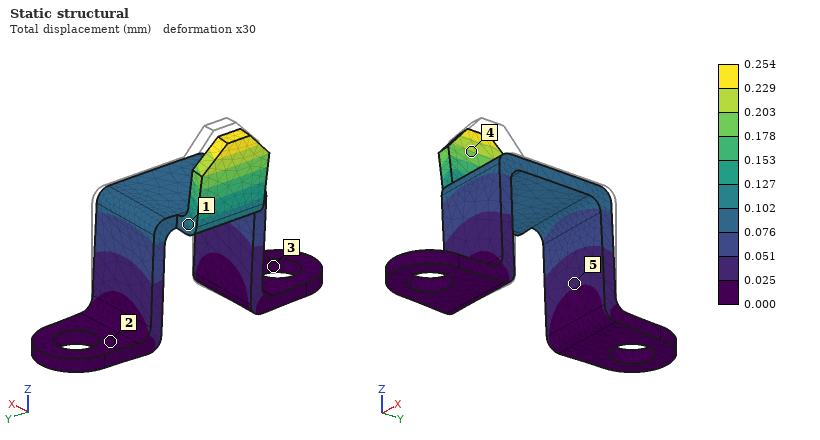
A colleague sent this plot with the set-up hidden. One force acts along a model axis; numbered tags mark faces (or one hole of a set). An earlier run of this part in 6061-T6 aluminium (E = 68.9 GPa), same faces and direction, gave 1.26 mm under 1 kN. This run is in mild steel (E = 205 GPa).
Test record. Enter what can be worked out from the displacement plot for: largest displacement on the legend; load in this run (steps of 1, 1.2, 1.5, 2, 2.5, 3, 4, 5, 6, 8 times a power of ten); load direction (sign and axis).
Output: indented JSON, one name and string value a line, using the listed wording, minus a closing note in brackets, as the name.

{
  "largest displacement on the legend": "0.254 mm",
  "load in this run": "600 N",
  "load direction": "-X"
}
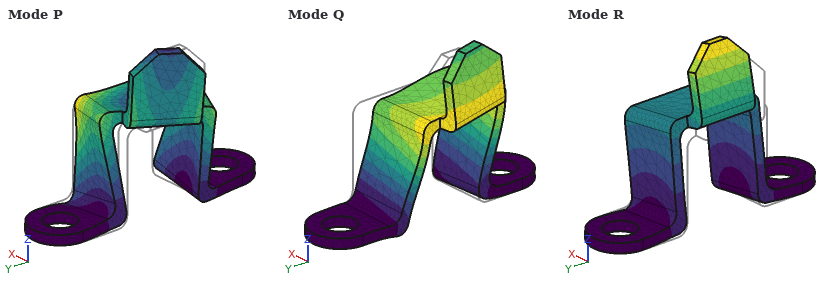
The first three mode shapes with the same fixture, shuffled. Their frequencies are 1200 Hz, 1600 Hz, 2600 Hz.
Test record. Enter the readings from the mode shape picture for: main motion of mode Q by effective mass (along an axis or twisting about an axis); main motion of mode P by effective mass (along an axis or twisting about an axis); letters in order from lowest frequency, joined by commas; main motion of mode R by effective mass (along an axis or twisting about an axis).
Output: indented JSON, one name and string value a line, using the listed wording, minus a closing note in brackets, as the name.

{
  "main motion of mode Q by effective mass": "along Y",
  "main motion of mode P by effective mass": "twisting about Z",
  "letters in order from lowest frequency, joined by commas": "R, Q, P",
  "main motion of mode R by effective mass": "along X"
}
